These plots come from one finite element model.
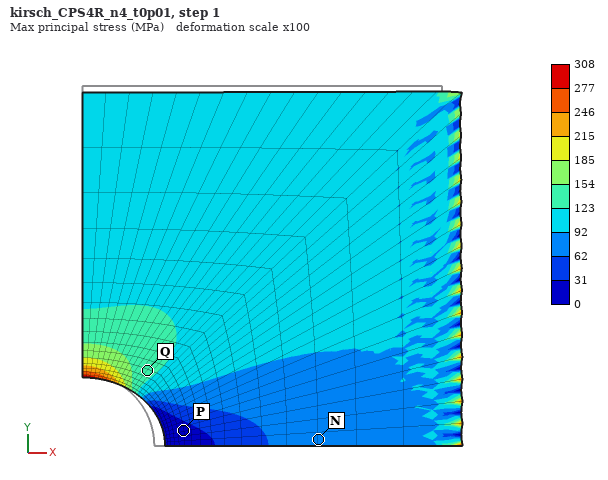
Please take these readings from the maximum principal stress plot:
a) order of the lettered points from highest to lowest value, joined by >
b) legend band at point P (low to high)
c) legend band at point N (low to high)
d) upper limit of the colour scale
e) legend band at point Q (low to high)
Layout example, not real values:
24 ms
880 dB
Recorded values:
Q > N > P
0 to 31 MPa
62 to 92 MPa
308 MPa
123 to 154 MPa
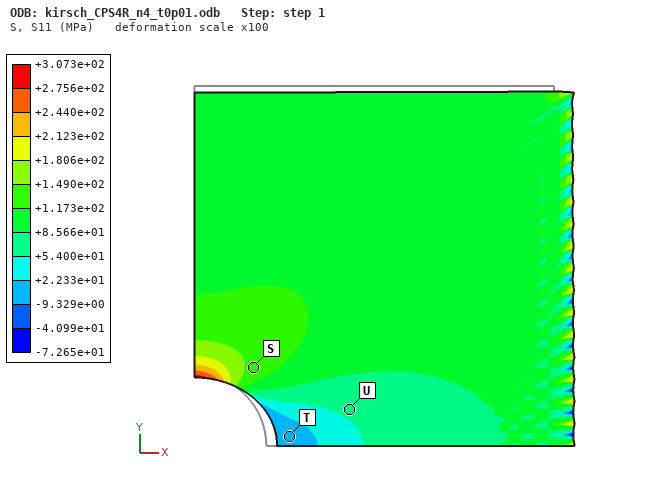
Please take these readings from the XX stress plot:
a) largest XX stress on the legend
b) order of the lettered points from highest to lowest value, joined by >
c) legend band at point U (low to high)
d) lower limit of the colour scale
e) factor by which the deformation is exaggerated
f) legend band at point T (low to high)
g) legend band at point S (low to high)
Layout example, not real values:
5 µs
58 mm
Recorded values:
+3.073e+02 MPa
S > U > T
+5.400e+01 to +8.566e+01 MPa
-7.265e+01 MPa
100
-9.329e+00 to +2.233e+01 MPa
+1.173e+02 to +1.490e+02 MPa
